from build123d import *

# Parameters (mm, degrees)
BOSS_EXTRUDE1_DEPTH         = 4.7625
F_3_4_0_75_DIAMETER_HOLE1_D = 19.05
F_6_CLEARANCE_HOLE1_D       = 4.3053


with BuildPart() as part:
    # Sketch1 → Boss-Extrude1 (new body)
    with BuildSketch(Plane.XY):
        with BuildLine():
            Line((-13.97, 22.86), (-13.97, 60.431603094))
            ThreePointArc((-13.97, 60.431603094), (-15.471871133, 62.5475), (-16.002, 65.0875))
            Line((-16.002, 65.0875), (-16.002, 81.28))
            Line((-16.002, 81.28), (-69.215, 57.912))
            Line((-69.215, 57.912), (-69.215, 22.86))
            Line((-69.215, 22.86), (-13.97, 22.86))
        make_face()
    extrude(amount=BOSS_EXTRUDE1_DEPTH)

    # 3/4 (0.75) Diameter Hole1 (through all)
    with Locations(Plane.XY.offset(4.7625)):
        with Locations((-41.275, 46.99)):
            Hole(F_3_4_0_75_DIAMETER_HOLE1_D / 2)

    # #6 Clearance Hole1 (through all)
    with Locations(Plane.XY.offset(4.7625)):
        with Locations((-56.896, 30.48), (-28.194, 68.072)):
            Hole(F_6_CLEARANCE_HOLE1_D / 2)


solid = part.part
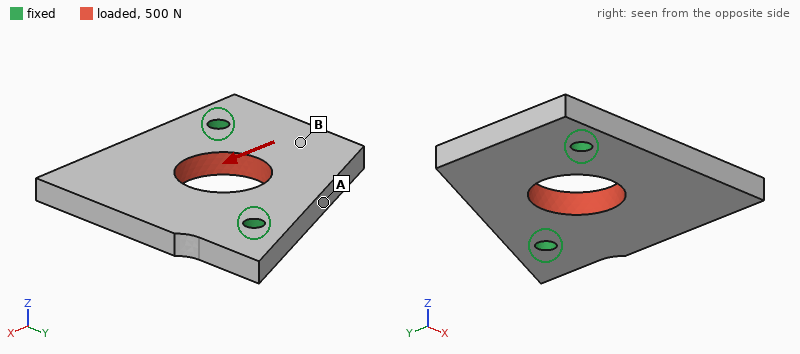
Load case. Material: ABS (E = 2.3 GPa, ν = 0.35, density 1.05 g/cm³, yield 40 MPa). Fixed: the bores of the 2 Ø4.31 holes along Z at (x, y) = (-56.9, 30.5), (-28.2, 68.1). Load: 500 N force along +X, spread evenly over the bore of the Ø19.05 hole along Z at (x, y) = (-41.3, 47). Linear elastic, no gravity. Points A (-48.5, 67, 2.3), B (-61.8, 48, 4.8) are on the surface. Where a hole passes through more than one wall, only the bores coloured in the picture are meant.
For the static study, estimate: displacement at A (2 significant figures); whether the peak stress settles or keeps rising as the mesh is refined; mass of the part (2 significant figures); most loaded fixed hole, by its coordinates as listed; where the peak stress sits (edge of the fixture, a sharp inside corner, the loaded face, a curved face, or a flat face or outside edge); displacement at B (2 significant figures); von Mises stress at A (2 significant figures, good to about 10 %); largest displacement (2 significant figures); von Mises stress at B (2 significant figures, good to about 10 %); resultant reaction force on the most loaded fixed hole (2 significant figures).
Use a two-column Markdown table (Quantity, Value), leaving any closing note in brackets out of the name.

| Quantity | Value |
|---|---|
| displacement at A | 30 µm |
| whether the peak stress settles or keeps rising as the mesh is refined | keeps rising |
| mass of the part | 11 g |
| most loaded fixed hole, by its coordinates as listed | (-56.9, 30.5) |
| where the peak stress sits | edge of the fixture |
| displacement at B | 30 µm |
| von Mises stress at A | 3.5 MPa |
| largest displacement | 45 µm |
| von Mises stress at B | 1.1 MPa |
| resultant reaction force on the most loaded fixed hole | 270 N |
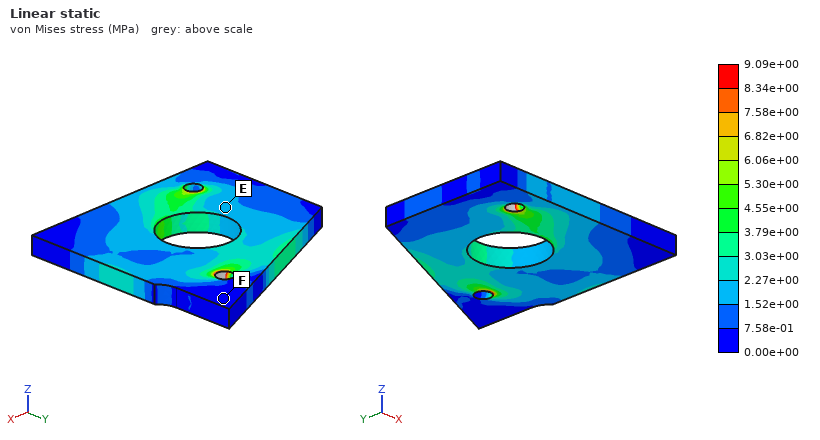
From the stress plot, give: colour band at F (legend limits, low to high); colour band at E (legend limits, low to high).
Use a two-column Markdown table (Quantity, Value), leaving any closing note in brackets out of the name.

| Quantity | Value |
|---|---|
| colour band at F | 0.00e+00 to 7.58e-01 MPa |
| colour band at E | 1.52e+00 to 2.27e+00 MPa |
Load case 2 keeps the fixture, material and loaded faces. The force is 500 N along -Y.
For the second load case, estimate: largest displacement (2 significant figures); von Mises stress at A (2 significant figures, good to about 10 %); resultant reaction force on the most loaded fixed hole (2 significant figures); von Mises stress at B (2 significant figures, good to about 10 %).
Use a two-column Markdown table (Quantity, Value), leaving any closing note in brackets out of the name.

| Quantity | Value |
|---|---|
| largest displacement | 42 µm |
| von Mises stress at A | 2.8 MPa |
| resultant reaction force on the most loaded fixed hole | 260 N |
| von Mises stress at B | 1.2 MPa |
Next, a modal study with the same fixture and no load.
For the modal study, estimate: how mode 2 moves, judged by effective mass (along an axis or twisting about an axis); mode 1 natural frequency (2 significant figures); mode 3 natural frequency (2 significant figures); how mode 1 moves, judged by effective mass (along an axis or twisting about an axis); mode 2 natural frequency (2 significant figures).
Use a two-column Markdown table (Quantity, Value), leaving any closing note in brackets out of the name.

| Quantity | Value |
|---|---|
| how mode 2 moves, judged by effective mass | along Z |
| mode 1 natural frequency | 990 Hz |
| mode 3 natural frequency | 3300 Hz |
| how mode 1 moves, judged by effective mass | along Z |
| mode 2 natural frequency | 1800 Hz |
